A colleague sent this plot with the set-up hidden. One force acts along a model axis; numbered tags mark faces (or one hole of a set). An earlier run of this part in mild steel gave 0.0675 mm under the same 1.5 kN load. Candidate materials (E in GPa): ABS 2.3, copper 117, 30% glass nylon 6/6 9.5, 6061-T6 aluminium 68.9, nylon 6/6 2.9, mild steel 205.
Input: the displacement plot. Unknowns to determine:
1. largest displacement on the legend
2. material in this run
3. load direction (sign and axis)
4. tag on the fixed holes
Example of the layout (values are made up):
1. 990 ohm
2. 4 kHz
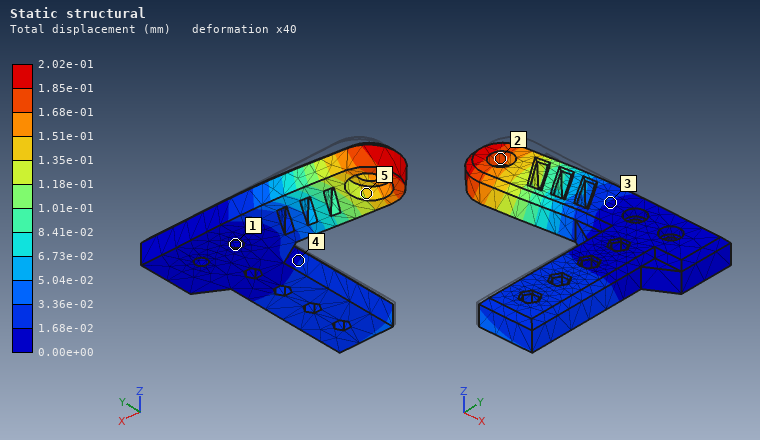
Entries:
1. 2.02e-01 mm
2. 6061-T6 aluminium
3. -Y
4. 1
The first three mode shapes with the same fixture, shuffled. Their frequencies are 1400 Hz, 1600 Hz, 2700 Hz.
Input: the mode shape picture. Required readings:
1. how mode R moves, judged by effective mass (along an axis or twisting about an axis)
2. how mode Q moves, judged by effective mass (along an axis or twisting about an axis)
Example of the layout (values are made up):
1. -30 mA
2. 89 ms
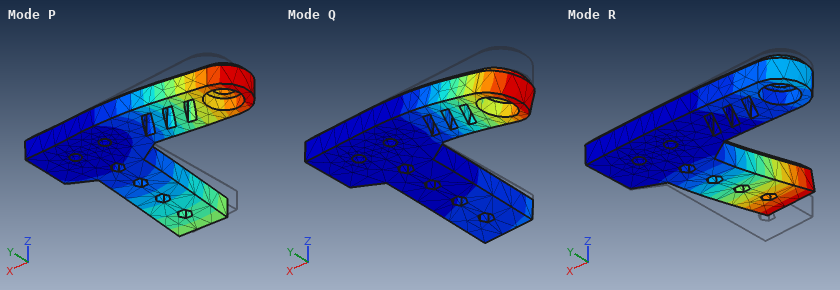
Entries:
1. along Z
2. along Z
